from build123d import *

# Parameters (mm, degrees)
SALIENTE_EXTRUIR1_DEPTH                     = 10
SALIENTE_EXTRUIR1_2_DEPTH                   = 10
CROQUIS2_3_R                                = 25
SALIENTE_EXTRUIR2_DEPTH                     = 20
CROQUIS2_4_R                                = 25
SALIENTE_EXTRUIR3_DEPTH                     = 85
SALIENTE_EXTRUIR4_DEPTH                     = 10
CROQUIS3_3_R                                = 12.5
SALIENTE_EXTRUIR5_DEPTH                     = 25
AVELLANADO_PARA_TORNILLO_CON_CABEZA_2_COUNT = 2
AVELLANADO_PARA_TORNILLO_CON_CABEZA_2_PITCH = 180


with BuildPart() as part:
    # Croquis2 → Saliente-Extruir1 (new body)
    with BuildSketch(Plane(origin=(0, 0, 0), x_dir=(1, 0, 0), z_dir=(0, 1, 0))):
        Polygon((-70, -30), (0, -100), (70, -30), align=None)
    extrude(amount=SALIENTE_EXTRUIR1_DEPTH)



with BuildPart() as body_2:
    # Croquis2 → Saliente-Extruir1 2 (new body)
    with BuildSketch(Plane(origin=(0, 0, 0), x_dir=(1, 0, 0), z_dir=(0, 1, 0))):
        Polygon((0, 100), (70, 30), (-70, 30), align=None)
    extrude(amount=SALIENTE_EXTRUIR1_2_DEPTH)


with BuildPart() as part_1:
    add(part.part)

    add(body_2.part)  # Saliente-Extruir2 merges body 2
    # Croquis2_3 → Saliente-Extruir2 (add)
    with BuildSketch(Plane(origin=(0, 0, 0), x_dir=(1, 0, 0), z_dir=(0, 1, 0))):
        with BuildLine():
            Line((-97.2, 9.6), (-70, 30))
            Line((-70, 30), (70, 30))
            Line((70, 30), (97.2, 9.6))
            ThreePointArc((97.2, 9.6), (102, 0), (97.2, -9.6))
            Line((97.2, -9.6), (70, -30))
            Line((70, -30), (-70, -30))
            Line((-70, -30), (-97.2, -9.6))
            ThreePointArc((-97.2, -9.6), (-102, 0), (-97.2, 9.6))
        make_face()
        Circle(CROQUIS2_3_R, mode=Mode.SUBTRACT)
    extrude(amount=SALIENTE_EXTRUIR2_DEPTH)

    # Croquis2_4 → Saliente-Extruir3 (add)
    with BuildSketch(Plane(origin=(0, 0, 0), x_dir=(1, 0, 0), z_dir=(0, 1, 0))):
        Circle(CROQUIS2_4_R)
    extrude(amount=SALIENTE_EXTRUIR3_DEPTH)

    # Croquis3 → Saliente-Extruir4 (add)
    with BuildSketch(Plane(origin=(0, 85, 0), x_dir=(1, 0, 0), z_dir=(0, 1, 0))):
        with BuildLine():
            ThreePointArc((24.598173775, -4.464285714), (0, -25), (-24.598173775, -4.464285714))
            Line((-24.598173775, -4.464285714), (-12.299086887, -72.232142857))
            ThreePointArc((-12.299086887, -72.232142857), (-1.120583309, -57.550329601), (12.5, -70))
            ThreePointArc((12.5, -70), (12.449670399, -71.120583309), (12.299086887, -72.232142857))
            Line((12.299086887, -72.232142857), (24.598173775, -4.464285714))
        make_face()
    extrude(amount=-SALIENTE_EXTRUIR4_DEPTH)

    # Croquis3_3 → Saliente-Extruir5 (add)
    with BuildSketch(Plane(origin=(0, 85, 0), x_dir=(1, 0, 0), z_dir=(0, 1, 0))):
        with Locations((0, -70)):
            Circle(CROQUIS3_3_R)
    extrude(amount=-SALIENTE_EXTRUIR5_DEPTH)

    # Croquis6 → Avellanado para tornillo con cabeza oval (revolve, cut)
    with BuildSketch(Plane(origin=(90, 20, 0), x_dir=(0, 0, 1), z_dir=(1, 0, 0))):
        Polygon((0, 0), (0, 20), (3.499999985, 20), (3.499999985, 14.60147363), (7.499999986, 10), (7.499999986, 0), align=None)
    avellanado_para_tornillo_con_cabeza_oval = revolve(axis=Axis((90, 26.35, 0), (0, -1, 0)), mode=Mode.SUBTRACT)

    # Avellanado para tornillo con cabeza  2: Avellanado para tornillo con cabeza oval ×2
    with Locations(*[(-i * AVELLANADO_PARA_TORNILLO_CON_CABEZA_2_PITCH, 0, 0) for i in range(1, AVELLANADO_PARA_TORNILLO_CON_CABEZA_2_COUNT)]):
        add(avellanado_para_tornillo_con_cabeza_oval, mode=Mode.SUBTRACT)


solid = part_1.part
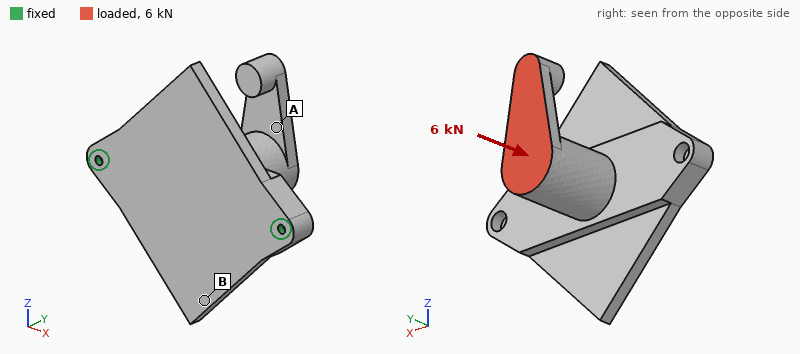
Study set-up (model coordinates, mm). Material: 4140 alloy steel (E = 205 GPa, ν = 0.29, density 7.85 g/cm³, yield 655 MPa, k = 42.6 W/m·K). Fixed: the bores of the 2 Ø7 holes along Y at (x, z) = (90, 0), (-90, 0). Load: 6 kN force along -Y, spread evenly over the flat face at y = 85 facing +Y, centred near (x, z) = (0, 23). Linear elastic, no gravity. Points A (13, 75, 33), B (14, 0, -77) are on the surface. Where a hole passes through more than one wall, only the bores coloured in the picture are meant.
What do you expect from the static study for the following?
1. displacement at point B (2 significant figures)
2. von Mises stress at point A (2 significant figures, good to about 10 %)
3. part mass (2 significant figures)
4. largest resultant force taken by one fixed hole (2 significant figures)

0.12 mm
68 MPa
3.6 kg
6.0 kN
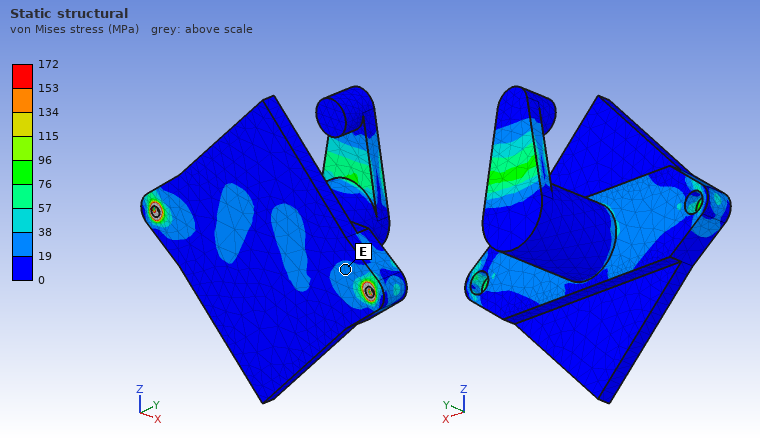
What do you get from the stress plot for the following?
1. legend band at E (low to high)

19 to 38 MPa
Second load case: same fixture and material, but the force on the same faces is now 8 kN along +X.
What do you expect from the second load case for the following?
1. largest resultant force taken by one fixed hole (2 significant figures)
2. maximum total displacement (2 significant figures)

5.6 kN
0.10 mm
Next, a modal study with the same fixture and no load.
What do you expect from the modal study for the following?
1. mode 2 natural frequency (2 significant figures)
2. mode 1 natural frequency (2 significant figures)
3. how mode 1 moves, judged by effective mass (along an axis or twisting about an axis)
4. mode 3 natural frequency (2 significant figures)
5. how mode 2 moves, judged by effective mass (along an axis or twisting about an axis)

1200 Hz
480 Hz
along Z
1800 Hz
along Y
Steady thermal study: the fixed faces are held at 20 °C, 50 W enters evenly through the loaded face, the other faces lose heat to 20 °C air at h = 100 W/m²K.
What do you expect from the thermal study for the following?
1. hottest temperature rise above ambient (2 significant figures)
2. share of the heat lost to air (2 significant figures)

39 K
93 %
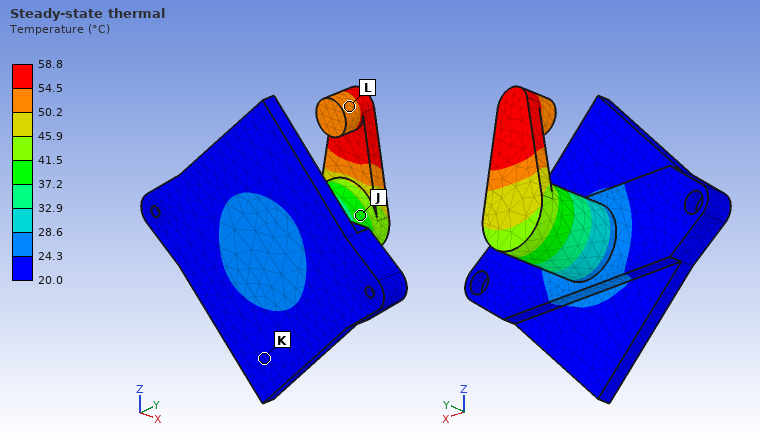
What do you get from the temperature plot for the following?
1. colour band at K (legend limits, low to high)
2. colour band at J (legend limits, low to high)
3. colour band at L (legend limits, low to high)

20.0 to 24.3 °C
37.2 to 41.5 °C
50.2 to 54.5 °C
